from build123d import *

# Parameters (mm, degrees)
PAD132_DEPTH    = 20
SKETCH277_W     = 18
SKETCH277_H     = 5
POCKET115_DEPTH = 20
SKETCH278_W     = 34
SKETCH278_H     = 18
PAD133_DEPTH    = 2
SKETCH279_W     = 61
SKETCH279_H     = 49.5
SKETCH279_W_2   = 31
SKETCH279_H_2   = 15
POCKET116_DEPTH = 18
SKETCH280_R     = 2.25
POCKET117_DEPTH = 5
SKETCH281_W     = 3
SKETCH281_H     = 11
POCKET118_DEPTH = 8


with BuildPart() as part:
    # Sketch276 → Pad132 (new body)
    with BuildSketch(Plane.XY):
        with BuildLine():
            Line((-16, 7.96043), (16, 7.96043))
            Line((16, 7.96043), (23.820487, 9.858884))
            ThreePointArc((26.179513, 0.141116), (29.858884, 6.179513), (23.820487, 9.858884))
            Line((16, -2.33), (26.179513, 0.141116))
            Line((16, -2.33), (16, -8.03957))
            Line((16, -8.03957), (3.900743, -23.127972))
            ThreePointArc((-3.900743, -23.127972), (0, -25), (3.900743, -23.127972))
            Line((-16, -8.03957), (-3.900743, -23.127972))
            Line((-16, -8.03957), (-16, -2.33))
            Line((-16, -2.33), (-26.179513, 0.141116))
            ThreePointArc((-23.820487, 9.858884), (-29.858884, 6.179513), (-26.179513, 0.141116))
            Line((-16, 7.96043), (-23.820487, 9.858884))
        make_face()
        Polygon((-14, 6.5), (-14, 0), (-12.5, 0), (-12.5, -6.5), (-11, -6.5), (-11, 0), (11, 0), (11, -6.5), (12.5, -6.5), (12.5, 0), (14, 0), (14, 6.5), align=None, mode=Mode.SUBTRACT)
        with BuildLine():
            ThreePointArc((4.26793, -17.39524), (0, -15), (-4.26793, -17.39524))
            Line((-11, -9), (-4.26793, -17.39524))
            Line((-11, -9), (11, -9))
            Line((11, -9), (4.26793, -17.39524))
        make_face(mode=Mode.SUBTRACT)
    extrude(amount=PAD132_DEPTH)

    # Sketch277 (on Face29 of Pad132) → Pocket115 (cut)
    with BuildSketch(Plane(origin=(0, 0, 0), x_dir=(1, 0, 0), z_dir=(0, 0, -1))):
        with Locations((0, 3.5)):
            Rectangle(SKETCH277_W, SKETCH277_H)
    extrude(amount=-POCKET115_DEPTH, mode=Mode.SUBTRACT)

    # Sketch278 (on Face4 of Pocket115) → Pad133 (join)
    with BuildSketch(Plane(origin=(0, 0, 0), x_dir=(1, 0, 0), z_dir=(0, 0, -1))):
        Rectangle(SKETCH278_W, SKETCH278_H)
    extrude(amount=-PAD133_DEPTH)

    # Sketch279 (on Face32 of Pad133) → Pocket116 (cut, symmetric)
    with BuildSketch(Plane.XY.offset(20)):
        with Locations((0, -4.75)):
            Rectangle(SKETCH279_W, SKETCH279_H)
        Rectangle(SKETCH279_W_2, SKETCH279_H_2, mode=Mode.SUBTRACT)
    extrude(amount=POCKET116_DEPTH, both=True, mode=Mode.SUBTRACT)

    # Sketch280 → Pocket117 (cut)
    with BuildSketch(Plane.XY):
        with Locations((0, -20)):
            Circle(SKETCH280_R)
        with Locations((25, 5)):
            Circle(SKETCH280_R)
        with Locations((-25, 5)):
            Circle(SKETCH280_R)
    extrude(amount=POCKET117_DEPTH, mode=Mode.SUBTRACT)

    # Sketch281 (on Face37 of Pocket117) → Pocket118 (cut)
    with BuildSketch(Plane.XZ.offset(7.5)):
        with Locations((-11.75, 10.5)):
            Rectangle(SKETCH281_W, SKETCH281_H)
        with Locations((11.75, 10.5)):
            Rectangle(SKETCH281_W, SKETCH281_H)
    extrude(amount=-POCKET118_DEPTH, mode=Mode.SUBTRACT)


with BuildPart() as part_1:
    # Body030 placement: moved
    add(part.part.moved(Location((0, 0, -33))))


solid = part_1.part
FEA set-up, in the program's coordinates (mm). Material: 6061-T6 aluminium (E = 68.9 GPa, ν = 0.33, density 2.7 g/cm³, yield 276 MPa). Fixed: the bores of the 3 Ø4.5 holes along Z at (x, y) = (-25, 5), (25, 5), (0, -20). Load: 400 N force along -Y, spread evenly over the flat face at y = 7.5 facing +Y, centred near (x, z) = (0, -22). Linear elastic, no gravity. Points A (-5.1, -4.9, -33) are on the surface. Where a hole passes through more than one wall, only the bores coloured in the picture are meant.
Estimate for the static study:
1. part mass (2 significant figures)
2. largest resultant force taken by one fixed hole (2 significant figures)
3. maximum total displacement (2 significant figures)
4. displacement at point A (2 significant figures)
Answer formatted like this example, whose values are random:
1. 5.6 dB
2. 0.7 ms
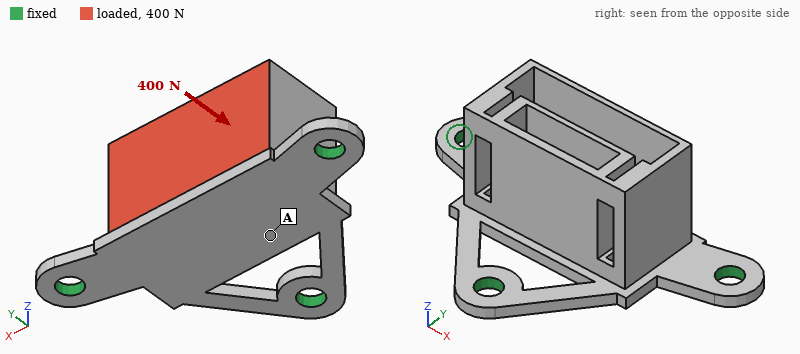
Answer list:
1. 13 g
2. 180 N
3. 0.40 mm
4. 0.060 mm
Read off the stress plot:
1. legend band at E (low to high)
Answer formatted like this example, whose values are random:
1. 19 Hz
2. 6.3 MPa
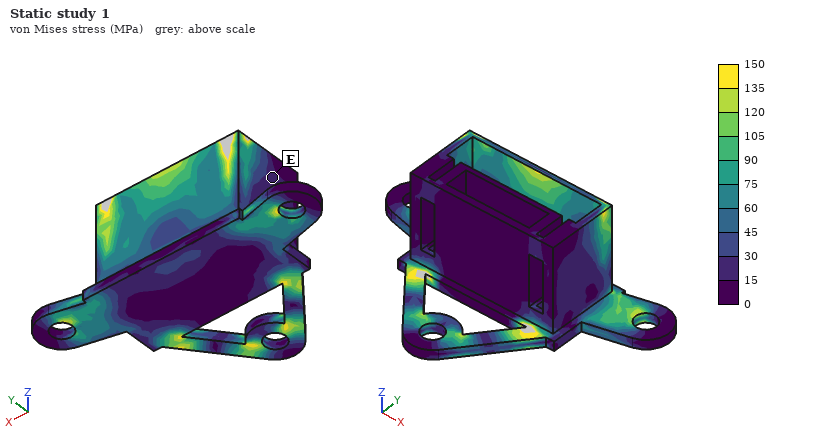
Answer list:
1. 15 to 30 MPa
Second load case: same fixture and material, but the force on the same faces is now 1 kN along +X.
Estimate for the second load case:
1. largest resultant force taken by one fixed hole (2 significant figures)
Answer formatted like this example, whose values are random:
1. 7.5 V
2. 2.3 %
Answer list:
1. 570 N
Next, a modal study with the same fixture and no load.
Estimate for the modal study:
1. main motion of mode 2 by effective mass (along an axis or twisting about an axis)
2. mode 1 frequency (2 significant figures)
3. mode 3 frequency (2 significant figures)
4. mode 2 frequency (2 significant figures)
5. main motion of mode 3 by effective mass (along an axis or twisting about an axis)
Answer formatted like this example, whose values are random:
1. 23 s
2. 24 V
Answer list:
1. along Z
2. 2900 Hz
3. 6000 Hz
4. 5500 Hz
5. along X
